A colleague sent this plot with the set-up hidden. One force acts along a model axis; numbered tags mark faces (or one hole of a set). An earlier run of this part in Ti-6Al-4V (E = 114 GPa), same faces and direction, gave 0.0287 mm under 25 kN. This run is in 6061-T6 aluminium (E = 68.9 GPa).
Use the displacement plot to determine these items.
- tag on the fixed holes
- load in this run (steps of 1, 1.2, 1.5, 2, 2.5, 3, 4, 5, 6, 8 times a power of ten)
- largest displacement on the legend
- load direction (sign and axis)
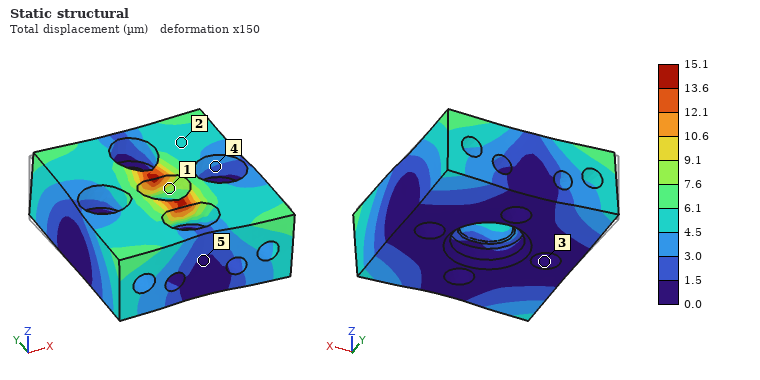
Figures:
3
8 kN
15.1 µm
-Y
